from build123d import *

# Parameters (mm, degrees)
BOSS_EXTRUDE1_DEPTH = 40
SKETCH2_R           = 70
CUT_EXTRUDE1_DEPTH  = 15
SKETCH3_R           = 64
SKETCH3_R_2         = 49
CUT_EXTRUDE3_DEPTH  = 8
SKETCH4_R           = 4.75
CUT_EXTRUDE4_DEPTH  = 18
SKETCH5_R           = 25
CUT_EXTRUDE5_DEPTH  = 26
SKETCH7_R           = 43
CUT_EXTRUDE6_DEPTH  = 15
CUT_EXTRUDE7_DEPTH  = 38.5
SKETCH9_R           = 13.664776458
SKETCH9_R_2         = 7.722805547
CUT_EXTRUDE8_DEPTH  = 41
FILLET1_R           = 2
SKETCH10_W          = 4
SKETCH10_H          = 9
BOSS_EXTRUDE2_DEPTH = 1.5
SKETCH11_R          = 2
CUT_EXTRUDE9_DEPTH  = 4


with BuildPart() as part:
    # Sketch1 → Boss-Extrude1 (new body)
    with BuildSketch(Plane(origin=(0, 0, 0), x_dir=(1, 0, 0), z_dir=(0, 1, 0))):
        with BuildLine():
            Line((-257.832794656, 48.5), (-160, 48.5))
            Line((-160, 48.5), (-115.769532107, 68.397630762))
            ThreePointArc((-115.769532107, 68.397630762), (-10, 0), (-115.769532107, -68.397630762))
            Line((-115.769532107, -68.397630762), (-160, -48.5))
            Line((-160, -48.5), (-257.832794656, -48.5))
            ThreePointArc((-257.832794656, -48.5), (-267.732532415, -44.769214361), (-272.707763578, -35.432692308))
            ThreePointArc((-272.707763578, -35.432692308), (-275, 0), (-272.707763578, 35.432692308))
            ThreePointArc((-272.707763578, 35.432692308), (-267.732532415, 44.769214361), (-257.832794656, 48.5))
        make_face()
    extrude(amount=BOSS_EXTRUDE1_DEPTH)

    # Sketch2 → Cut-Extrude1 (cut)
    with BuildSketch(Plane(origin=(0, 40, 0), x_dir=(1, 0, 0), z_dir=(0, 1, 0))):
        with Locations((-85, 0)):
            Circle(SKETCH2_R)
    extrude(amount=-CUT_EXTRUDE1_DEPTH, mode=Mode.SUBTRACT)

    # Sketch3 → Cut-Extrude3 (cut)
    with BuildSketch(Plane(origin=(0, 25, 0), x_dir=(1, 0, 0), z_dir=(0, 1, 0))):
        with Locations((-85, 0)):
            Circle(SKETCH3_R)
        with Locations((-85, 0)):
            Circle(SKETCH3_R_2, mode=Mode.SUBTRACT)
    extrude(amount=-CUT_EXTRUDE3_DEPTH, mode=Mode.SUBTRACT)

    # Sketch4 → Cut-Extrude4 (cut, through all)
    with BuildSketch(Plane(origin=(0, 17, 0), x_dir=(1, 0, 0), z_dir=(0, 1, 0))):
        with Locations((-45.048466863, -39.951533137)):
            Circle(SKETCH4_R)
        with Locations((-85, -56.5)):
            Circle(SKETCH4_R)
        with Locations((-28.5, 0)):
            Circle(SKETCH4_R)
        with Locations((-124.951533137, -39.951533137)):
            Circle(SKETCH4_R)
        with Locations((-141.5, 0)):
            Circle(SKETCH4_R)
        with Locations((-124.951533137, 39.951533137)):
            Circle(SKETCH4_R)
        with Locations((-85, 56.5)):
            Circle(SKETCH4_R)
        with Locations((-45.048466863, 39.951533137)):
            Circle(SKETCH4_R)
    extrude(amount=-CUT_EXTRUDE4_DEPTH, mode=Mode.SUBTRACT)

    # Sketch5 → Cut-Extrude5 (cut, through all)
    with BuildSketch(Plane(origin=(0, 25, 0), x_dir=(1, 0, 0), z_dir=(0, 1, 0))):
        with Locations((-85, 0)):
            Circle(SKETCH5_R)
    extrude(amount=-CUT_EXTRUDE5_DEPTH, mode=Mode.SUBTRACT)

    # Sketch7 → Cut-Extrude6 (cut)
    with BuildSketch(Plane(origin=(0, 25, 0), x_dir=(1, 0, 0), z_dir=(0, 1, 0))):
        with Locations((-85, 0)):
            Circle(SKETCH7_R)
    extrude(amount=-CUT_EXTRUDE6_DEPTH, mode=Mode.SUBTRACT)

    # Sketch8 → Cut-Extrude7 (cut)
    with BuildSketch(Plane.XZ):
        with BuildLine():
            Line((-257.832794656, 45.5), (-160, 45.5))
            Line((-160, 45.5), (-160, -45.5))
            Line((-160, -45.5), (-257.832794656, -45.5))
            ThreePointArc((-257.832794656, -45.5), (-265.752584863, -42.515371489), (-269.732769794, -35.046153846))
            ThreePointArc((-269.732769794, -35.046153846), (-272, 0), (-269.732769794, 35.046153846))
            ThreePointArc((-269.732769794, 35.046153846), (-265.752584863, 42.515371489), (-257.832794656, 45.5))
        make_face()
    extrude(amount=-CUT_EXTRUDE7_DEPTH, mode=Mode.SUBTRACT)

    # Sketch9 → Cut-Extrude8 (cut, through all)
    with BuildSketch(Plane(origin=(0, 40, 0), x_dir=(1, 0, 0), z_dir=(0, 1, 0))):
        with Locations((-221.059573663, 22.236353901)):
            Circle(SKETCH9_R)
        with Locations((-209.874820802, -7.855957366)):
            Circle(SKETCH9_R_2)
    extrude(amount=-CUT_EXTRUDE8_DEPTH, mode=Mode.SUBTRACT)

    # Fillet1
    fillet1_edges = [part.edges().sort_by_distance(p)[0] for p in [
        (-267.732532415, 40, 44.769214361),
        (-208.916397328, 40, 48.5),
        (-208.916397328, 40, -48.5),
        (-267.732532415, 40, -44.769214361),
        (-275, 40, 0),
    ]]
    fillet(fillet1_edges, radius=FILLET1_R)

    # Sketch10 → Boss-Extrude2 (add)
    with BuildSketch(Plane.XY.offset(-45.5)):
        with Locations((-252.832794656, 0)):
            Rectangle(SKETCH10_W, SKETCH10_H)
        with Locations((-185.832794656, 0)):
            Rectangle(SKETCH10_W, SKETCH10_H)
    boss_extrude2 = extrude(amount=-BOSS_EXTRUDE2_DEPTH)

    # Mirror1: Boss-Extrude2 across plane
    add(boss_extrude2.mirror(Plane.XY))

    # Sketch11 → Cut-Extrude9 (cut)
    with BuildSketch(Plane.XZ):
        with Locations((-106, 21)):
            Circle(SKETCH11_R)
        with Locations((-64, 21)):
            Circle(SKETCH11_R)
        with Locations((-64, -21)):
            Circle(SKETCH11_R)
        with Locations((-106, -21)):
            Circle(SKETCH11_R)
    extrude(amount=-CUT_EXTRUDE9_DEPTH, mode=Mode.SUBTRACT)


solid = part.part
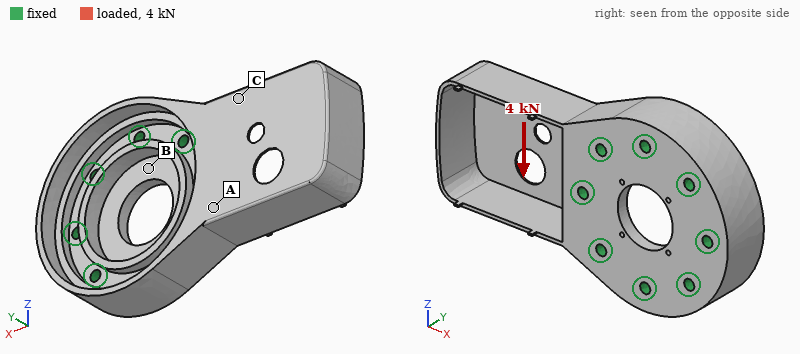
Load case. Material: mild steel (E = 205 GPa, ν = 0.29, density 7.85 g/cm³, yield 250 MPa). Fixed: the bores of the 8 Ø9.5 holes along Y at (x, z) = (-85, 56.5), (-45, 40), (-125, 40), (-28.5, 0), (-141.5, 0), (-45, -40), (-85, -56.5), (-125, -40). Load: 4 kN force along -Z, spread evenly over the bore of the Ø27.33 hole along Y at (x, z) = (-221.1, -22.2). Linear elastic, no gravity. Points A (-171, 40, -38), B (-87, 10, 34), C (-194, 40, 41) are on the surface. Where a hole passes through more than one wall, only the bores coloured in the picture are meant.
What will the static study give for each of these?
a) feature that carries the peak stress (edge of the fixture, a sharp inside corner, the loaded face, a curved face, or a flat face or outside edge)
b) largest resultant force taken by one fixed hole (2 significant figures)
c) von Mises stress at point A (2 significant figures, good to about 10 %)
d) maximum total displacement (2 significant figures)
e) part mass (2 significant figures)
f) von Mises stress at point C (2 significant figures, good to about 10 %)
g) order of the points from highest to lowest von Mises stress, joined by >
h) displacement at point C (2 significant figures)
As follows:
the loaded face
2.4 kN
54 MPa
0.12 mm
3.1 kg
38 MPa
A > C > B
0.027 mm
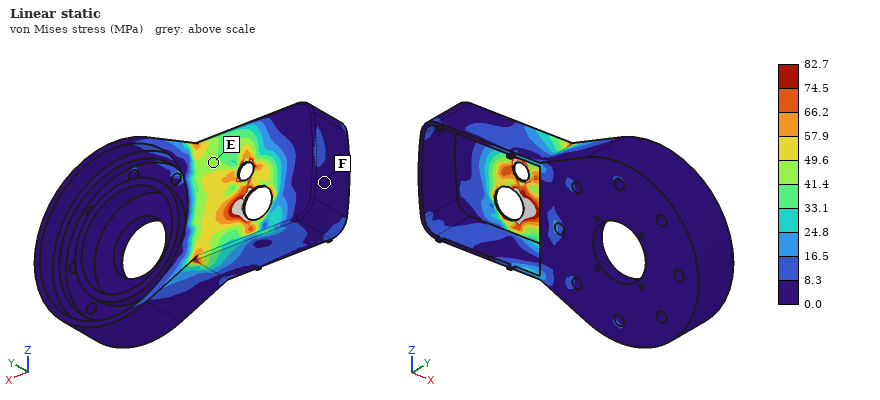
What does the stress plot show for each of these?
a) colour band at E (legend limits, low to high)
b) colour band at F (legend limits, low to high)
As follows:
41.4 to 49.6 MPa
0.0 to 8.3 MPa
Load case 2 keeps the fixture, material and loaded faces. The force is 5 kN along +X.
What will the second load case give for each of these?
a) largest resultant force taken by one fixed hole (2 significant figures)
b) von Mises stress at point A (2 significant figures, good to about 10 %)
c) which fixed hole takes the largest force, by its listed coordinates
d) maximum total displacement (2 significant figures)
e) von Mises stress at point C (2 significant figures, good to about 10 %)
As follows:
2.3 kN
49 MPa
(-125, -40)
98 µm
10.0 MPa
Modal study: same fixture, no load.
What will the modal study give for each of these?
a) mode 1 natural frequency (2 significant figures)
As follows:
1100 Hz
